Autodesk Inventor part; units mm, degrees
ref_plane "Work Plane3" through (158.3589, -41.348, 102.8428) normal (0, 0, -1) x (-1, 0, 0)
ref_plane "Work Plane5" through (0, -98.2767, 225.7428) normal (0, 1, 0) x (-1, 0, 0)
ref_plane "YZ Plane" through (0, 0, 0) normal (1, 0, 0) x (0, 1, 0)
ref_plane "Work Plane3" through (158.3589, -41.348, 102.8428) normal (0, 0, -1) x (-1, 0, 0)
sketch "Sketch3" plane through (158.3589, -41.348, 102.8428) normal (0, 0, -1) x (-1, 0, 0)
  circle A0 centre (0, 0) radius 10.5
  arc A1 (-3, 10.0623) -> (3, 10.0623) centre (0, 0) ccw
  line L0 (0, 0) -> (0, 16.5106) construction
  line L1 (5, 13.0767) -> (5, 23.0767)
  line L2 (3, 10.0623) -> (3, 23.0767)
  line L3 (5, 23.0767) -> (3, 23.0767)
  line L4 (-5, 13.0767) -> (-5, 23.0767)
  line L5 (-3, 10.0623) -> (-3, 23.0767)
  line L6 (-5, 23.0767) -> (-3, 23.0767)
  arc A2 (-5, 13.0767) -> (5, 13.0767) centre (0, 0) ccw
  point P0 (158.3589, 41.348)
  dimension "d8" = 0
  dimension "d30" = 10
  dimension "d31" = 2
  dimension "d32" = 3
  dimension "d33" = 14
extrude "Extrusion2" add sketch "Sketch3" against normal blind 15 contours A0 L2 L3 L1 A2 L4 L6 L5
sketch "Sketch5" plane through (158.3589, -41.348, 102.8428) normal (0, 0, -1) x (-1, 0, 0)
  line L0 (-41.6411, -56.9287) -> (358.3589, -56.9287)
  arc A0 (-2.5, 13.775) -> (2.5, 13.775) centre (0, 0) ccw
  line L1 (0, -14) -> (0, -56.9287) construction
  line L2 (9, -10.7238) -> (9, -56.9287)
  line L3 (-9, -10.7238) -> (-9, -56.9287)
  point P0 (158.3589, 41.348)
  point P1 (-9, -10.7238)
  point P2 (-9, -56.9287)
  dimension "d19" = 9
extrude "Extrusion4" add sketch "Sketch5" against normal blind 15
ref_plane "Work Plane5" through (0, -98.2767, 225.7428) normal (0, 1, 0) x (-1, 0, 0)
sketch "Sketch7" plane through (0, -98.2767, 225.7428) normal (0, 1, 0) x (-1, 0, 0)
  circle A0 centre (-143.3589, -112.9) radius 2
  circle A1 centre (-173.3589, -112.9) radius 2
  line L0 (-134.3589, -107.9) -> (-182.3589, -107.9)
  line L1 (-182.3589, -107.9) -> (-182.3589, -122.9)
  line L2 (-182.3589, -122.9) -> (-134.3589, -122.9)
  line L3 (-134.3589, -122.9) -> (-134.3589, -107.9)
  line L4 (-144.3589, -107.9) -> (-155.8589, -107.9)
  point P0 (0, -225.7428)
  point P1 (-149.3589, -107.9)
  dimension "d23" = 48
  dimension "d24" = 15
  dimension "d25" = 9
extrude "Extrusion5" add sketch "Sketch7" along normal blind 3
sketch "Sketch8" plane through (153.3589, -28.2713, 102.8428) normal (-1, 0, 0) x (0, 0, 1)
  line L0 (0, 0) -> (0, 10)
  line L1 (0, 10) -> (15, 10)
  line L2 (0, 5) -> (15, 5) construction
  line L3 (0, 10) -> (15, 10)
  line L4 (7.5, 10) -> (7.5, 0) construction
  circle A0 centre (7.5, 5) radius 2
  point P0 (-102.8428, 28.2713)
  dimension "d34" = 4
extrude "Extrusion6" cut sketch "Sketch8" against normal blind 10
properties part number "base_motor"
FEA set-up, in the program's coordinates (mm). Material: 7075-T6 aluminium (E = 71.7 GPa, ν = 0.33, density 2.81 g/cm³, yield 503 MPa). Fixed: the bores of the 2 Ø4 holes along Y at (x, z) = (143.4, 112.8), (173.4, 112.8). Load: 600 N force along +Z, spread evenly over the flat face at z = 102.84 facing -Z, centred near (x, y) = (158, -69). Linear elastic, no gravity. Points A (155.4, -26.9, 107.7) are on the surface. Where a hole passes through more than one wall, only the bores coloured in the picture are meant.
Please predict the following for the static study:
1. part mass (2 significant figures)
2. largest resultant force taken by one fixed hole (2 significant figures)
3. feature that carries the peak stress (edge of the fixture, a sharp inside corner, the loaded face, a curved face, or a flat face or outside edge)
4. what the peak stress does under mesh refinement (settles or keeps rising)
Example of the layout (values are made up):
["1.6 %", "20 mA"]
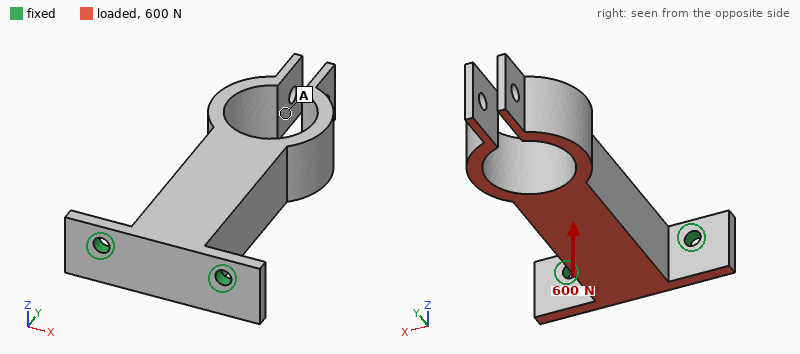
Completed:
["49 g", "350 N", "edge of the fixture", "keeps rising"]
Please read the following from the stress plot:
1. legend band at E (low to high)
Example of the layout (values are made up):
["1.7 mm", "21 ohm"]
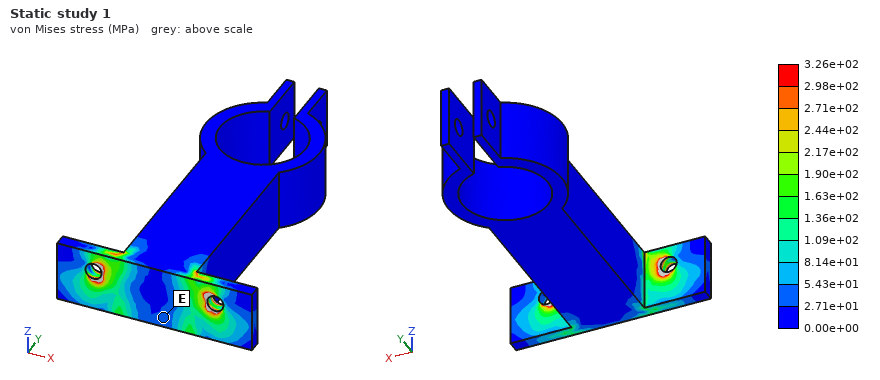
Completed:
["2.71e+01 to 5.43e+01 MPa"]
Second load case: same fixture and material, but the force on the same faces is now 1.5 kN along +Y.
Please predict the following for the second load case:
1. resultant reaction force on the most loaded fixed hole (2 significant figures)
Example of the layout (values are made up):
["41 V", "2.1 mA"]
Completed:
["780 N"]
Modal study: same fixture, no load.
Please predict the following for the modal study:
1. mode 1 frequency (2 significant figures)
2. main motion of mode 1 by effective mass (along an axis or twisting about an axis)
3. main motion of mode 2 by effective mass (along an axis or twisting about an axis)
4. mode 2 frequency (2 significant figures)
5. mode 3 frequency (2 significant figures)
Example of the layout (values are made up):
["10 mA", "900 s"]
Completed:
["760 Hz", "along Z", "along X", "1700 Hz", "2600 Hz"]
